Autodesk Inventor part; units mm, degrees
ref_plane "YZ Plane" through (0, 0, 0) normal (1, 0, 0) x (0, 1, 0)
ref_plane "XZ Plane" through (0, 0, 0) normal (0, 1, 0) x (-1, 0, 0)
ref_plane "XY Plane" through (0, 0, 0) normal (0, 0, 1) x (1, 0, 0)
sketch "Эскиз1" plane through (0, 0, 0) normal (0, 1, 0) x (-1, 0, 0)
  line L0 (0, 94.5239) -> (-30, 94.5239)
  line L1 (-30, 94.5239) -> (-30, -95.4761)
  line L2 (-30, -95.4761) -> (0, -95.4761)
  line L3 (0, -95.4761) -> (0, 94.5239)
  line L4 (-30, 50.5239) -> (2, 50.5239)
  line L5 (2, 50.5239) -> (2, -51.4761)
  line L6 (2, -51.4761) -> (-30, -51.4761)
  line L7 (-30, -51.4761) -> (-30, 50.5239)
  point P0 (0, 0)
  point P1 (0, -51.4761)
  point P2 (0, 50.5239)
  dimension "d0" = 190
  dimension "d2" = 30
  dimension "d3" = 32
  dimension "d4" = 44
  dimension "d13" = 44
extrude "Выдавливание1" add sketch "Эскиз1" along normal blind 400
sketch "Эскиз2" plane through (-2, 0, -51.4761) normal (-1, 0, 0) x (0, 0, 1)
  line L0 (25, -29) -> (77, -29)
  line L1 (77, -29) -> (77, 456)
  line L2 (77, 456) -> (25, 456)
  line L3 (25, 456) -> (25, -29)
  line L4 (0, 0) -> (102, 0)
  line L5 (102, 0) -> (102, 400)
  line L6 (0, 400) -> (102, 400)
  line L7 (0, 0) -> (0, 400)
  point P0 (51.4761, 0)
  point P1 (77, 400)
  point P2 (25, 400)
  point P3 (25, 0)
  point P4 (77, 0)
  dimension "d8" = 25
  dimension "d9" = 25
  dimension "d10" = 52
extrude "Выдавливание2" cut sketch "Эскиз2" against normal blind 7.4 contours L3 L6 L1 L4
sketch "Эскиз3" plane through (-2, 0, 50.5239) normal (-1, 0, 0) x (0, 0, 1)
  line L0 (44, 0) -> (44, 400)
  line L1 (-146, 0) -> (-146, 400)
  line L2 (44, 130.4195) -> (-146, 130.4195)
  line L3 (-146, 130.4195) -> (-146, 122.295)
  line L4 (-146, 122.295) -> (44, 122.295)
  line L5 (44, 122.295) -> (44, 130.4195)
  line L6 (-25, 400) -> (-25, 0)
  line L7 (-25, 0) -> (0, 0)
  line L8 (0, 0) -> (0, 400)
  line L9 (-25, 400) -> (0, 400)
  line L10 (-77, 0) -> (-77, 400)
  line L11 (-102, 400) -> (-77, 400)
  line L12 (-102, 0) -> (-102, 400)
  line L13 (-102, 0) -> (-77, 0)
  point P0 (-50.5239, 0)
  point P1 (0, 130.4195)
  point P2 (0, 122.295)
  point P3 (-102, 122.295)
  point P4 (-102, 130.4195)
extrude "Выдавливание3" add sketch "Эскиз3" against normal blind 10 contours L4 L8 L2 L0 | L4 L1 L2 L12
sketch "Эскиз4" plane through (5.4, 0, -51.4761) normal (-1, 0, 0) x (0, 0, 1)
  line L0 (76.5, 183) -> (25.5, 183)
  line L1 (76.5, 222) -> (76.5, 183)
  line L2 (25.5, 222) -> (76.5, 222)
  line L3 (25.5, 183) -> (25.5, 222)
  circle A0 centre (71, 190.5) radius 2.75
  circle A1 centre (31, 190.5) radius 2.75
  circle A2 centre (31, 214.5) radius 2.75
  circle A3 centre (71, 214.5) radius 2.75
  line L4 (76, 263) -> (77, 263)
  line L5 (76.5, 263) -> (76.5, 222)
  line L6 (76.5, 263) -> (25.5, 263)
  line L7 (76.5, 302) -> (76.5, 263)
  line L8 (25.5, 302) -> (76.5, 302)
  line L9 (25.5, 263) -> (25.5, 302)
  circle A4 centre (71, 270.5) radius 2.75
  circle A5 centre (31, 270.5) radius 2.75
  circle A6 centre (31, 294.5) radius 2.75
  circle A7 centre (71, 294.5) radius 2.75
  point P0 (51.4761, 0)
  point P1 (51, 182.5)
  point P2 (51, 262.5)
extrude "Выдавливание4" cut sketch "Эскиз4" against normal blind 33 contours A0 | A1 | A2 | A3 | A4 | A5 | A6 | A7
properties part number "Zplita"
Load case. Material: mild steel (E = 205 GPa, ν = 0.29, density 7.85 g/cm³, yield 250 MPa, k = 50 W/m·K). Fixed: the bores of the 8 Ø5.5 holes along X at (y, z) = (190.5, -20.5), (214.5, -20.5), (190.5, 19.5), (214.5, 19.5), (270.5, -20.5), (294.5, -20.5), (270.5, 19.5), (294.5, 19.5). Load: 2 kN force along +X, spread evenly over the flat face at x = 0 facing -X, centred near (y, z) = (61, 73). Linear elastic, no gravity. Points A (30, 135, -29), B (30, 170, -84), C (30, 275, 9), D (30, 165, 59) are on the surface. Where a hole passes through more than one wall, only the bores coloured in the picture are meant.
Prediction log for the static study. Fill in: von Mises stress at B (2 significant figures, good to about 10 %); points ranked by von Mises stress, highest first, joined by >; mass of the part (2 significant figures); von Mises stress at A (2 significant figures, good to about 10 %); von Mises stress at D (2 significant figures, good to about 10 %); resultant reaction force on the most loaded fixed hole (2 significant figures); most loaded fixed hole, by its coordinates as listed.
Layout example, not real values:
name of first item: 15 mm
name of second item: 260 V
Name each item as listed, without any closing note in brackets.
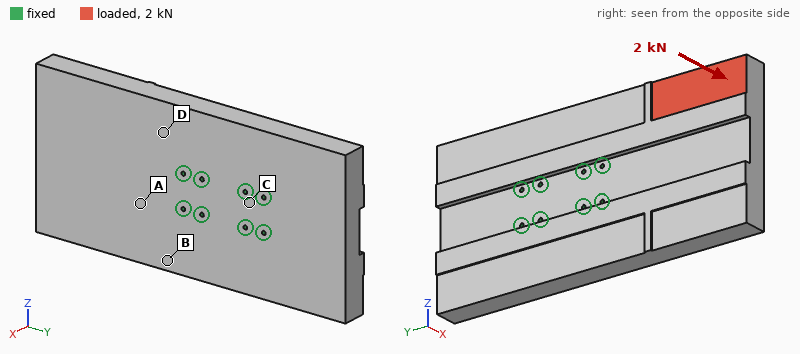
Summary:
von Mises stress at B: 4.9 MPa
points ranked by von Mises stress, highest first, joined by >: D > A > B > C
mass of the part: 17 kg
von Mises stress at A: 6.3 MPa
von Mises stress at D: 8.2 MPa
resultant reaction force on the most loaded fixed hole: 3.9 kN
most loaded fixed hole, by its coordinates as listed: (190.5, 19.5)
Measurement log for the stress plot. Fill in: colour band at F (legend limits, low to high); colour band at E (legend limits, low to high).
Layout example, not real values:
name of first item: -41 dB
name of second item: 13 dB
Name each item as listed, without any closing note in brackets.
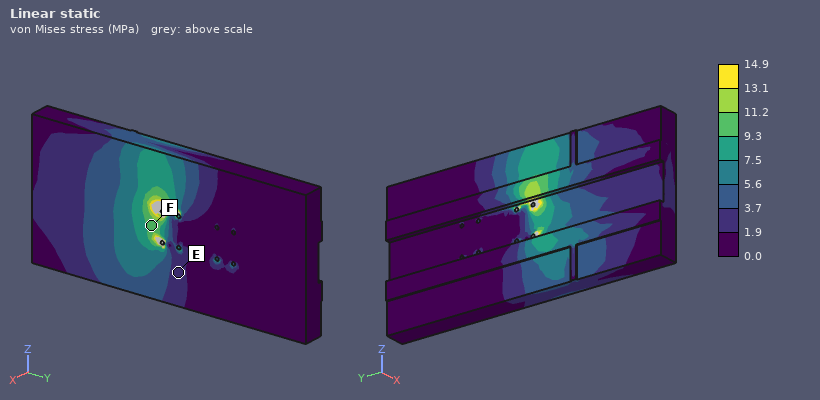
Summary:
colour band at F: 9.3 to 11.2 MPa
colour band at E: 1.9 to 3.7 MPa
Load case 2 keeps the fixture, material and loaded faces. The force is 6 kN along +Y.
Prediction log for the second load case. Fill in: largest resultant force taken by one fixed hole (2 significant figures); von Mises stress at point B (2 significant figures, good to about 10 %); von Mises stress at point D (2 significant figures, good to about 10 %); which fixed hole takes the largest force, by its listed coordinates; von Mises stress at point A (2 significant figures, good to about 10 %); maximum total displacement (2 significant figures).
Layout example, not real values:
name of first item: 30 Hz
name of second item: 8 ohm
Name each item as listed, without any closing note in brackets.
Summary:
largest resultant force taken by one fixed hole: 3.3 kN
von Mises stress at point B: 3.6 MPa
von Mises stress at point D: 1.2 MPa
which fixed hole takes the largest force, by its listed coordinates: (190.5, 19.5)
von Mises stress at point A: 2.8 MPa
maximum total displacement: 28 µm
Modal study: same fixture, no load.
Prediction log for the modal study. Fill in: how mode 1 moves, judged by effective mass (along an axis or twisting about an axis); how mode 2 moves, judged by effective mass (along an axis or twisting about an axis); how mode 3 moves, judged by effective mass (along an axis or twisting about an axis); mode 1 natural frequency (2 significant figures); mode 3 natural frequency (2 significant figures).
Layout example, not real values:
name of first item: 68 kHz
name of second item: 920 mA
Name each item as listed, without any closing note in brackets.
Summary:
how mode 1 moves, judged by effective mass: along X
how mode 2 moves, judged by effective mass: twisting about Y
how mode 3 moves, judged by effective mass: along X
mode 1 natural frequency: 560 Hz
mode 3 natural frequency: 1500 Hz
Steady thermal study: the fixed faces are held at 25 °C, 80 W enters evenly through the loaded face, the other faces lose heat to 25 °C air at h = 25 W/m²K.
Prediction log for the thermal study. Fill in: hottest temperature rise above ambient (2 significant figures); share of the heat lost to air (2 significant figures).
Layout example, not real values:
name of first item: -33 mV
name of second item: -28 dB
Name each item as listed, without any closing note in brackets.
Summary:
hottest temperature rise above ambient: 44 K
share of the heat lost to air: 50 %
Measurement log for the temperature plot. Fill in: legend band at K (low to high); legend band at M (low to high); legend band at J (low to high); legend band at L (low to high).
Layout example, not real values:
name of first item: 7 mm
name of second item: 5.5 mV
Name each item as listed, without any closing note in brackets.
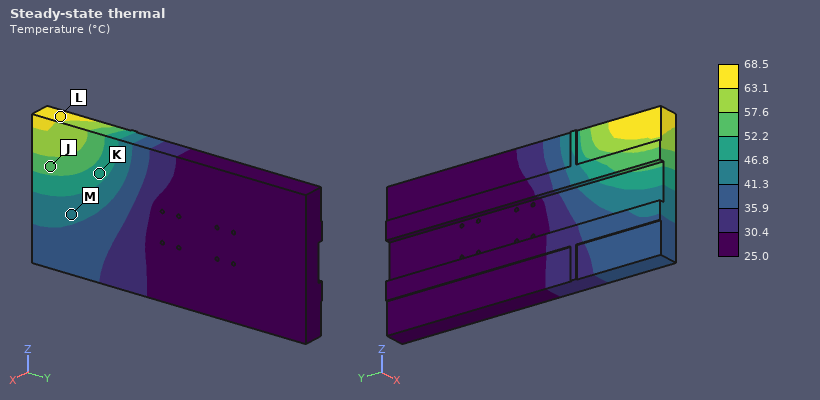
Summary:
legend band at K: 46.8 to 52.2 °C
legend band at M: 41.3 to 46.8 °C
legend band at J: 52.2 to 57.6 °C
legend band at L: 63.1 to 68.5 °C
